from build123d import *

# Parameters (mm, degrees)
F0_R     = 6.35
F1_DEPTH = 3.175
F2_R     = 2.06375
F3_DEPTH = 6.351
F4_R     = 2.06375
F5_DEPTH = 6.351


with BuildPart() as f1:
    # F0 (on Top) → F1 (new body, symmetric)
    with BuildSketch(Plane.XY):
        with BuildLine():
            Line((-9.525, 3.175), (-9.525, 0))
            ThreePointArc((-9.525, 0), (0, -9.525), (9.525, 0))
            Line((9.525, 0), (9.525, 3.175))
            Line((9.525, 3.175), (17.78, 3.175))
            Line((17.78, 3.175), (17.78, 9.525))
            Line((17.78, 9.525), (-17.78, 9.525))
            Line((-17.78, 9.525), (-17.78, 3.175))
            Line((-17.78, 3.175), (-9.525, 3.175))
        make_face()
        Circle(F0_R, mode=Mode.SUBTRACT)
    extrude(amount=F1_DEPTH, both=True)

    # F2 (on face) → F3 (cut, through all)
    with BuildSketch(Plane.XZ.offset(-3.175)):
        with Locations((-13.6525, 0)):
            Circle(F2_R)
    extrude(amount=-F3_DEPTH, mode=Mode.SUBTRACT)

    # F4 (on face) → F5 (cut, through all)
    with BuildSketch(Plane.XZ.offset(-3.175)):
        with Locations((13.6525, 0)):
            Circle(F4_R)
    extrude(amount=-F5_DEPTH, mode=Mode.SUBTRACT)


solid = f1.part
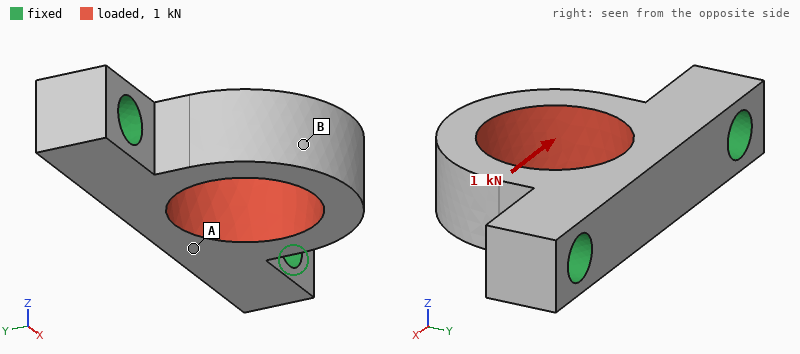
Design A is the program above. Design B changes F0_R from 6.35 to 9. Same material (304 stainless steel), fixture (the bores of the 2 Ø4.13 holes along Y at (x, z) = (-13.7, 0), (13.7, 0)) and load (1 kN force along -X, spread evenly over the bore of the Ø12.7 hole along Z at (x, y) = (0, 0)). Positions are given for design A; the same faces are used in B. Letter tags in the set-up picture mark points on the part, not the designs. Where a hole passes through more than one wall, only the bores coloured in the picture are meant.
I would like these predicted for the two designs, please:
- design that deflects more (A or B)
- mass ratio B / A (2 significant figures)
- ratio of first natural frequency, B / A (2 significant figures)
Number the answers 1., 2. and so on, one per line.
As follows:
1. B
2. 0.54
3. 0.35
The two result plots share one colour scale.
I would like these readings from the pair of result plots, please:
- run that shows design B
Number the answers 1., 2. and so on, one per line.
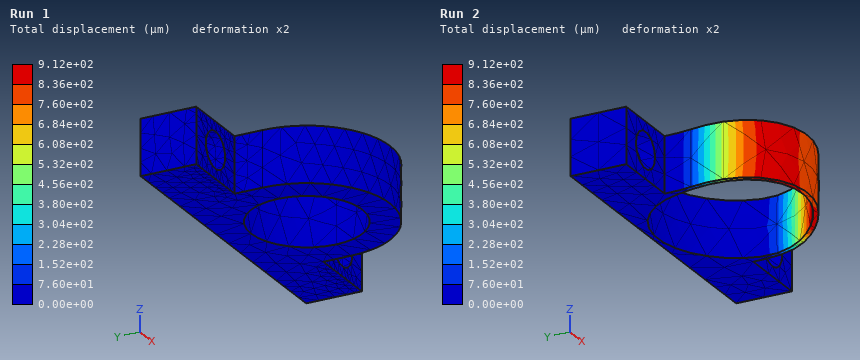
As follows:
1. Run 2
